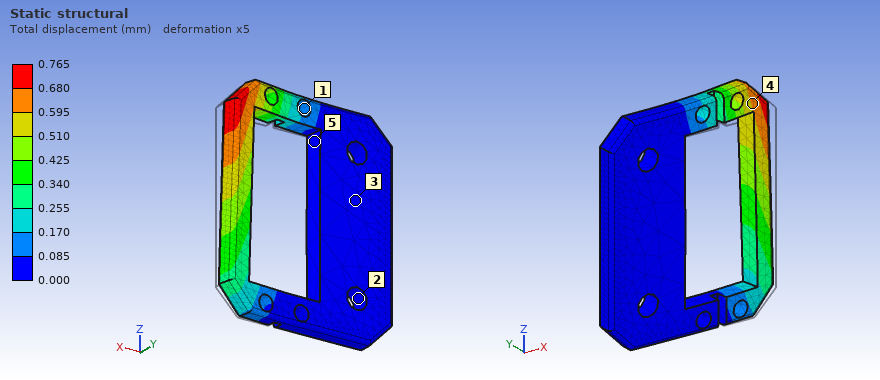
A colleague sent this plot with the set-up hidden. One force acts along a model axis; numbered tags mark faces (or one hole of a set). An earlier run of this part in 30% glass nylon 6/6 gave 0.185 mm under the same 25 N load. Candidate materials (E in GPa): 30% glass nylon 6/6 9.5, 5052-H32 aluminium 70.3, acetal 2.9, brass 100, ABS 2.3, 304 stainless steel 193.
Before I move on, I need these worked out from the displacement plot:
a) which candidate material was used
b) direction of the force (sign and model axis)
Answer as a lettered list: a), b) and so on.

a) ABS
b) +Y
